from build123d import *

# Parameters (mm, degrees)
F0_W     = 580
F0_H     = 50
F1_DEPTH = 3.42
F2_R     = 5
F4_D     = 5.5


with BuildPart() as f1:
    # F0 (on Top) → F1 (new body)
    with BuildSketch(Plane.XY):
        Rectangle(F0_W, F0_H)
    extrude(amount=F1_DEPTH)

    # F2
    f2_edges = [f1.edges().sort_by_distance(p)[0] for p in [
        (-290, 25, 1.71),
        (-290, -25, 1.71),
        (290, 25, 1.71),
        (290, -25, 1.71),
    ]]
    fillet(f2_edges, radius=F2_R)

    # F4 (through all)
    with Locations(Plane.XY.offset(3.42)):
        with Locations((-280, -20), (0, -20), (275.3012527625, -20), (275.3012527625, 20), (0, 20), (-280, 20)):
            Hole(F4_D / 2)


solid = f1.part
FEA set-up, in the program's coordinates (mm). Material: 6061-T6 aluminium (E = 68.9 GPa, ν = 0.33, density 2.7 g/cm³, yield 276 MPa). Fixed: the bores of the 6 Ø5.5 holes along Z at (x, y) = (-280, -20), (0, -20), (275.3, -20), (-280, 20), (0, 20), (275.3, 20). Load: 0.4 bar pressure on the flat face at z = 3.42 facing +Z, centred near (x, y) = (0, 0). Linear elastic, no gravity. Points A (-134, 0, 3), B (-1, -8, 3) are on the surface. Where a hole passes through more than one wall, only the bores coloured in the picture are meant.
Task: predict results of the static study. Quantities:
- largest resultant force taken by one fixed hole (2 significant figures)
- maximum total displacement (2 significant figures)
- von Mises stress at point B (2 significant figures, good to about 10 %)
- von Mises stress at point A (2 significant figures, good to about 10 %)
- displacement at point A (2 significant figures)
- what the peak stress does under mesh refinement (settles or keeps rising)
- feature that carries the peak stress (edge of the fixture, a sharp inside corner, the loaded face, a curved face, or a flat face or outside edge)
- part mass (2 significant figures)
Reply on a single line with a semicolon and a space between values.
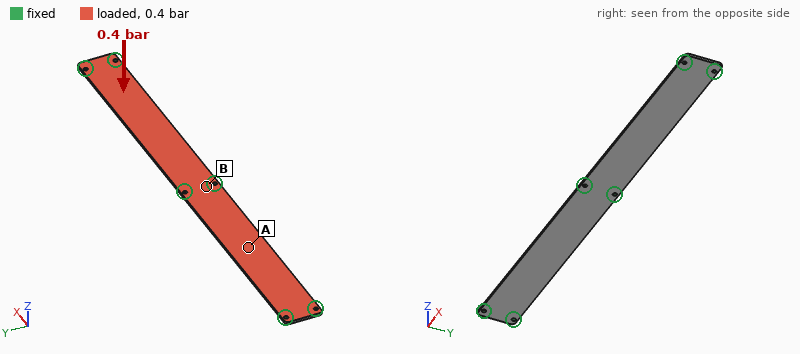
280 N; 2.7 mm; 100 MPa; 64 MPa; 2.7 mm; keeps rising; edge of the fixture; 270 g
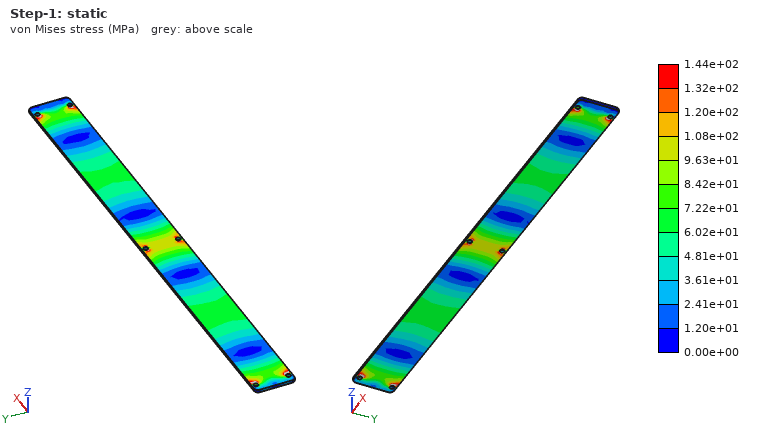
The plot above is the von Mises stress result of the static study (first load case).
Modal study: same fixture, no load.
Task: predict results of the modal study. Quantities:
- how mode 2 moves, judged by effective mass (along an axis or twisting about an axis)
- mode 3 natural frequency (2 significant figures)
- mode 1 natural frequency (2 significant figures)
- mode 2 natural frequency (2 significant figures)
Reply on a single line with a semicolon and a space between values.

along Z; 620 Hz; 230 Hz; 240 Hz
